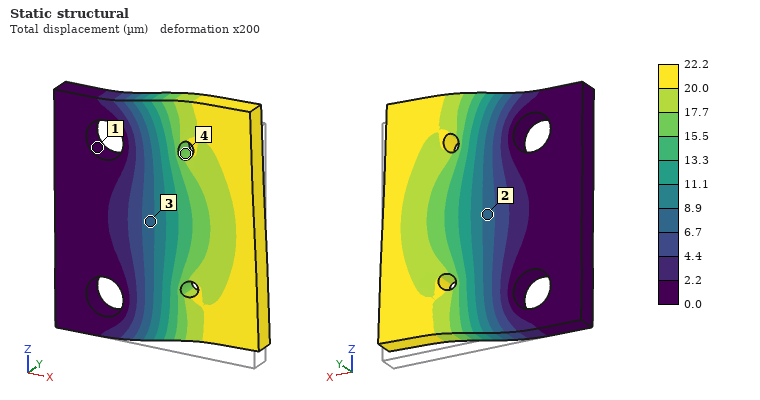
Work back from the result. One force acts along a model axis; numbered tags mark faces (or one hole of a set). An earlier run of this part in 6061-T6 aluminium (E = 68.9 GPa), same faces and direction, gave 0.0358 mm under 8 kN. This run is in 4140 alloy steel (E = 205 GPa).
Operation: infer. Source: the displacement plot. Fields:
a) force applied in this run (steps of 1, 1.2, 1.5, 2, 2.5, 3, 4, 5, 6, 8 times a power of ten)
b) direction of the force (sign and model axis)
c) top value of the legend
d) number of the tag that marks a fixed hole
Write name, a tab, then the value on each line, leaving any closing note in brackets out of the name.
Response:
force applied in this run	15 kN
direction of the force	+Z
top value of the legend	22.2 µm
number of the tag that marks a fixed hole	1
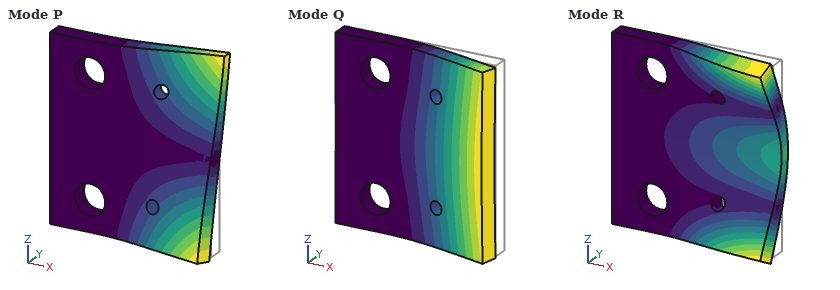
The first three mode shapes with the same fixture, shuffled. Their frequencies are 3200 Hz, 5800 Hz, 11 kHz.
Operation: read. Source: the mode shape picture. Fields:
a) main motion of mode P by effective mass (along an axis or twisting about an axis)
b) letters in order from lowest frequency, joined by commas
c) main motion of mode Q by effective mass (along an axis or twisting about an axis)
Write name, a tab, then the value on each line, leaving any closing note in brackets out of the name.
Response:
main motion of mode P by effective mass	twisting about X
letters in order from lowest frequency, joined by commas	Q, P, R
main motion of mode Q by effective mass	along Y
